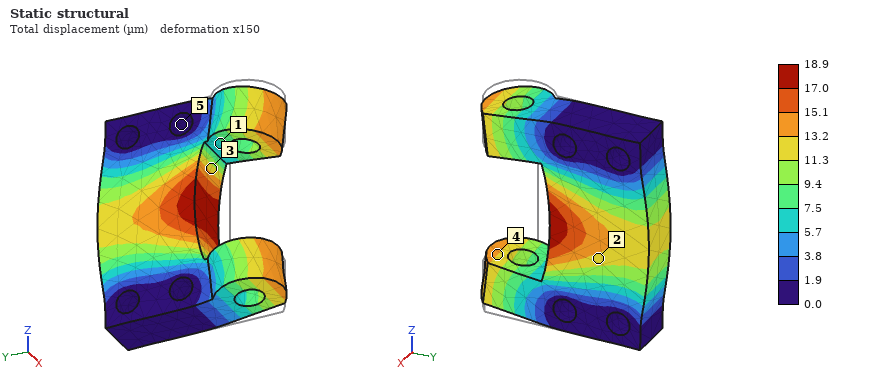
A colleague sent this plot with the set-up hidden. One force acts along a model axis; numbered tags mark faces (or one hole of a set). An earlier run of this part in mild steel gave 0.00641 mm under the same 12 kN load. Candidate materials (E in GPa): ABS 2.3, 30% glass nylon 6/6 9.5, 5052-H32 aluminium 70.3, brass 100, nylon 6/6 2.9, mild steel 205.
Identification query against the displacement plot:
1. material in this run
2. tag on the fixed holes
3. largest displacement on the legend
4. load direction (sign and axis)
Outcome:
5052-H32 aluminium
5
18.9 µm
+Y
